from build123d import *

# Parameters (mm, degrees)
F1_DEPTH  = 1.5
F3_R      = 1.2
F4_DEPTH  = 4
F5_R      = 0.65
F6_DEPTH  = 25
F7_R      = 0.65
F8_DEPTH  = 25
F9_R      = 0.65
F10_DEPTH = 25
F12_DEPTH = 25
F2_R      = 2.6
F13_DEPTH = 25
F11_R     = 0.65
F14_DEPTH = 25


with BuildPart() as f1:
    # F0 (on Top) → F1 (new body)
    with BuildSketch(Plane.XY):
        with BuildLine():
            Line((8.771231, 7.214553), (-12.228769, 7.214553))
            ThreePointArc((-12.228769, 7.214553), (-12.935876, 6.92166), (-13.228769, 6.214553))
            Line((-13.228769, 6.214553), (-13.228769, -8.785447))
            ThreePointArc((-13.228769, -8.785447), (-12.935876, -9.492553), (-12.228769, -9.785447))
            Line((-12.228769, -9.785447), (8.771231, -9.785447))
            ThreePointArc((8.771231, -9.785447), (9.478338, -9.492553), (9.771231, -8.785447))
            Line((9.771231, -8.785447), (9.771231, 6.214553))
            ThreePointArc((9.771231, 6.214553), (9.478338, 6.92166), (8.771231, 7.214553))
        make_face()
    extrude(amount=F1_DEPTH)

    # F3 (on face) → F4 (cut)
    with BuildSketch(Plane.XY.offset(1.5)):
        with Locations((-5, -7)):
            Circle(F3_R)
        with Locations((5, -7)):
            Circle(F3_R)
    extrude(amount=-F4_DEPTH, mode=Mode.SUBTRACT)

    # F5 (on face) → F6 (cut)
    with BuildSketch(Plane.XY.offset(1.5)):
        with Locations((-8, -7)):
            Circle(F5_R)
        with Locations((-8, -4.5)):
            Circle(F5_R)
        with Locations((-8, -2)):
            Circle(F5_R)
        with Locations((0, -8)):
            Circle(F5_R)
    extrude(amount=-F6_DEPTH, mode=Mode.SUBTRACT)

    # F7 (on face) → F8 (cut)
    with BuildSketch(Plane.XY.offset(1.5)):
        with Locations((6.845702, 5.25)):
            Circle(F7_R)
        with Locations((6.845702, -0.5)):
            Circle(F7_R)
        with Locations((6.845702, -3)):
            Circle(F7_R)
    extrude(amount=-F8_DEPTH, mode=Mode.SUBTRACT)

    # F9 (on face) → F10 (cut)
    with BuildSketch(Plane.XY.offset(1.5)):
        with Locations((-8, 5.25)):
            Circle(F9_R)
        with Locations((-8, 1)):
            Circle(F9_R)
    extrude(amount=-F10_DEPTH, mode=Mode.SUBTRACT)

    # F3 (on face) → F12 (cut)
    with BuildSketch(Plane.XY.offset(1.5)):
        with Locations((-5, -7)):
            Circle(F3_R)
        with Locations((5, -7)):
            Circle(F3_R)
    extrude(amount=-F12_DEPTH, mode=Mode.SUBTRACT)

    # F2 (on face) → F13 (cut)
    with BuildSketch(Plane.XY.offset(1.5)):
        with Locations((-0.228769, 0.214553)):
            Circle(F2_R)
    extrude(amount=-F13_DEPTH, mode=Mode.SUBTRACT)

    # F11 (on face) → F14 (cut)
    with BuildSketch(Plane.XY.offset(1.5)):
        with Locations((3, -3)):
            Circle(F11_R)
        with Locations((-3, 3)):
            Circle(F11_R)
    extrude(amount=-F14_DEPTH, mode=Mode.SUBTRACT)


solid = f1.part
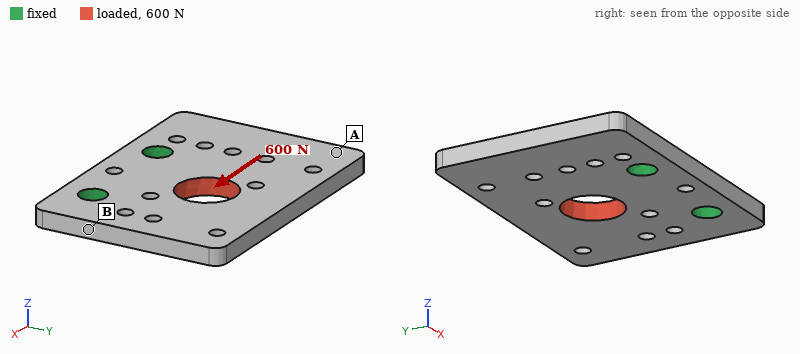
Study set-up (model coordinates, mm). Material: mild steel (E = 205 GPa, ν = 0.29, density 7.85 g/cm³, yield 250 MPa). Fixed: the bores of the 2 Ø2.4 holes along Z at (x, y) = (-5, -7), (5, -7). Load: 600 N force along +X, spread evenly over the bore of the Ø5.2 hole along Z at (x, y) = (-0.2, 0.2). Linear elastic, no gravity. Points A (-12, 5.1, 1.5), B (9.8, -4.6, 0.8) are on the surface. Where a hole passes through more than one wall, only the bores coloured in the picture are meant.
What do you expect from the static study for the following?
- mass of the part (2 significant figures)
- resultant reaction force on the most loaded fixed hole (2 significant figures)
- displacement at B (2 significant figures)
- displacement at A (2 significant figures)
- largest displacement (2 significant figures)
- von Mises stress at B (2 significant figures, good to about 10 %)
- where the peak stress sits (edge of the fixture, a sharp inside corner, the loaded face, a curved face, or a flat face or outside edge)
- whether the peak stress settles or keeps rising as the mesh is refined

4.1 g
440 N
2.4 µm
6.7 µm
7.5 µm
33 MPa
edge of the fixture
keeps rising
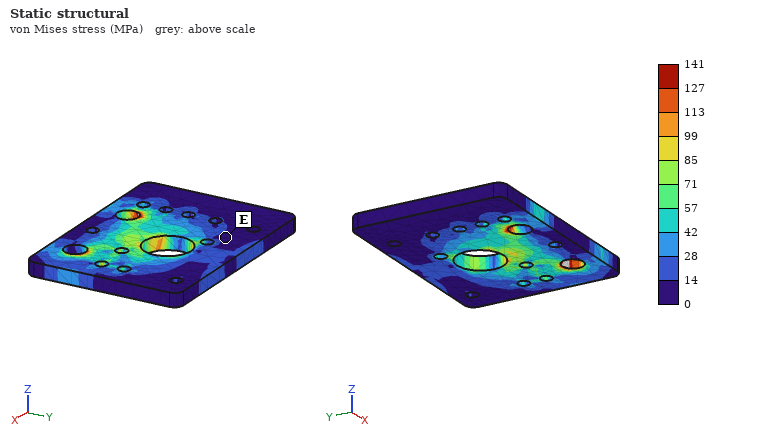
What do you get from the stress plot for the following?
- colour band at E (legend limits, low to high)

0 to 14 MPa
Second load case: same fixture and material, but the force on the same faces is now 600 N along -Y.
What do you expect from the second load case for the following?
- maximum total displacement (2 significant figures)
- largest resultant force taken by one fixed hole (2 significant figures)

2.2 µm
320 N
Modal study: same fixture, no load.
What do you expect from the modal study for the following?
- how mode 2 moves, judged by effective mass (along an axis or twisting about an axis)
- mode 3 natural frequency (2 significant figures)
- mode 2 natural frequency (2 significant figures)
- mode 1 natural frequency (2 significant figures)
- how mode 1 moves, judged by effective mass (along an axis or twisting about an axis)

twisting about Y
17 kHz
8900 Hz
5800 Hz
along Z
